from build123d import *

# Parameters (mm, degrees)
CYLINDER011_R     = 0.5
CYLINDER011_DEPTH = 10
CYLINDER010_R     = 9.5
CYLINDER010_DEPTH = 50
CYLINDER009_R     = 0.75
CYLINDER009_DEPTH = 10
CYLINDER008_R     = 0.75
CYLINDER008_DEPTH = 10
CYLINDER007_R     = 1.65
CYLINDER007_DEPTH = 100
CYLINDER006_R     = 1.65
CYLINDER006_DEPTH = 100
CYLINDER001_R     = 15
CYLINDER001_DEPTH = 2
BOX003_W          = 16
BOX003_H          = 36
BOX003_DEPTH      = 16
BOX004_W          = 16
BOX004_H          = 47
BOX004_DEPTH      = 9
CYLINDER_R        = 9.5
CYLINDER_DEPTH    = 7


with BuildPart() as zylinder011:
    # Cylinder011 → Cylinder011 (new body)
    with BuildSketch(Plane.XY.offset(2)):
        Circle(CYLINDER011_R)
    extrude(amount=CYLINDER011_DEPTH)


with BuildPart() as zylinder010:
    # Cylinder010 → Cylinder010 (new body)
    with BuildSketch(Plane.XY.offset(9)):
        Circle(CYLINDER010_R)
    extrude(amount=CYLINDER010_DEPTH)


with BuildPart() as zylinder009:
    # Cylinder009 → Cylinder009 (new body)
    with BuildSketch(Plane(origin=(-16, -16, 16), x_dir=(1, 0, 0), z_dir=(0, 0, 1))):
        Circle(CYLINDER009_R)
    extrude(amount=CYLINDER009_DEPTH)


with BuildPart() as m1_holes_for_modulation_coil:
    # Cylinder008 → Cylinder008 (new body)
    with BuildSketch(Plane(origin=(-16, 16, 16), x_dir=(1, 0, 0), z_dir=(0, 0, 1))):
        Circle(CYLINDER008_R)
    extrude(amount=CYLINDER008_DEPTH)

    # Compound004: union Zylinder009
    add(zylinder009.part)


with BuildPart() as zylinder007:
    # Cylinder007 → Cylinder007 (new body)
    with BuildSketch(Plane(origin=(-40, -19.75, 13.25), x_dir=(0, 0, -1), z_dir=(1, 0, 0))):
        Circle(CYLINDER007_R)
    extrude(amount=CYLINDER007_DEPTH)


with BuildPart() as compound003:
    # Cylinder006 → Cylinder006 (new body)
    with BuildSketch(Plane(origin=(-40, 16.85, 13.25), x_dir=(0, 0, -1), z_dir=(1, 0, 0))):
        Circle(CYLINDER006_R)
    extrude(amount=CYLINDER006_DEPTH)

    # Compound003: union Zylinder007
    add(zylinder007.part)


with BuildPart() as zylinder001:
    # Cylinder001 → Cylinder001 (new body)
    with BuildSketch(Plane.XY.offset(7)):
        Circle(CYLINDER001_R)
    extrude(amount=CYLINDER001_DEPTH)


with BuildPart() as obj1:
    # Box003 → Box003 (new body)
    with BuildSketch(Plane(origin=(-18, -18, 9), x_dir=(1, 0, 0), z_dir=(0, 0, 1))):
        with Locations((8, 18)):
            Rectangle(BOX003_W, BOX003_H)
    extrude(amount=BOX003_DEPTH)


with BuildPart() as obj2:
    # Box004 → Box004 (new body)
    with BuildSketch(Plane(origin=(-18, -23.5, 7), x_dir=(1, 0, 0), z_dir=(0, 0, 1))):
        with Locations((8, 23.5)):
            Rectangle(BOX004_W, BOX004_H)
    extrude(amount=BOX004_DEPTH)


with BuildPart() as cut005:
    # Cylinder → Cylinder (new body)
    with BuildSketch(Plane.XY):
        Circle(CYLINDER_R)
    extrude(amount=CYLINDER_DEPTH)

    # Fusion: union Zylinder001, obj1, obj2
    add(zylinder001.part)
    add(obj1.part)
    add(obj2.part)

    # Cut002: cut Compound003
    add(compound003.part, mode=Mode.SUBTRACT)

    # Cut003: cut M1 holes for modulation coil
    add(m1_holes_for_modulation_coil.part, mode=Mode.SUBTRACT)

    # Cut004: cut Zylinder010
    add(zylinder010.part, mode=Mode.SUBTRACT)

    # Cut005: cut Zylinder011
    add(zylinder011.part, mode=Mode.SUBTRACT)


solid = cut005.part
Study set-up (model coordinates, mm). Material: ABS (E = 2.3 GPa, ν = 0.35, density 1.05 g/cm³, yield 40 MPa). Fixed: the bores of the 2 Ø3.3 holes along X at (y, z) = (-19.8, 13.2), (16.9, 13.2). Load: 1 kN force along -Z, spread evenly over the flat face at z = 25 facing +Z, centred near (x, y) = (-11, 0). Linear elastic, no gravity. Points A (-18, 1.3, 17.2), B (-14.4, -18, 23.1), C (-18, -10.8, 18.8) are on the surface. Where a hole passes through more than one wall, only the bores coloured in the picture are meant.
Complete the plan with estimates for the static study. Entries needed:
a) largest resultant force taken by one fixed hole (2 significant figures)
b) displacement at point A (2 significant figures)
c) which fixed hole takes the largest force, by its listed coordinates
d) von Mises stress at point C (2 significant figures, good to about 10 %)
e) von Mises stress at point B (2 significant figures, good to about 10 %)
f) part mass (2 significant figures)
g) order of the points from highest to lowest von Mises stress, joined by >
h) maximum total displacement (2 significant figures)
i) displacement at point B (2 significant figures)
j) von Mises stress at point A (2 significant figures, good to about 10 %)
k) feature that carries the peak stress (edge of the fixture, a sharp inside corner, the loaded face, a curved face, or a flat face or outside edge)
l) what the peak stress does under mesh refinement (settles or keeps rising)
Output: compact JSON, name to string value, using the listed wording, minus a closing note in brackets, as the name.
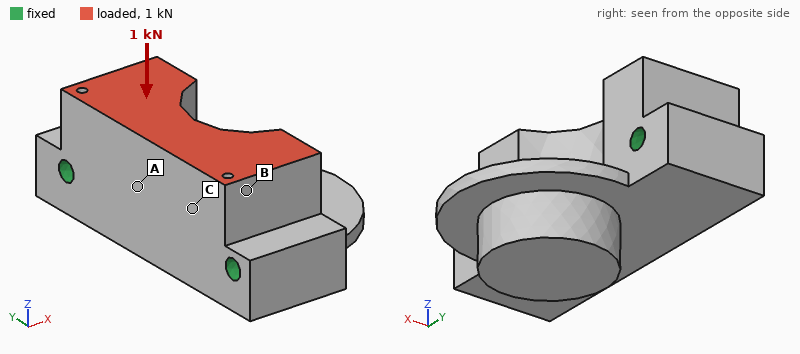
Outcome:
{"largest resultant force taken by one fixed hole": "550 N", "displacement at point A": "57 µm", "which fixed hole takes the largest force, by its listed coordinates": "(16.9, 13.2)", "von Mises stress at point C": "4.2 MPa", "von Mises stress at point B": "2.3 MPa", "part mass": "13 g", "order of the points from highest to lowest von Mises stress, joined by >": "C > B > A", "maximum total displacement": "66 µm", "displacement at point B": "28 µm", "von Mises stress at point A": "1.4 MPa", "feature that carries the peak stress": "edge of the fixture", "what the peak stress does under mesh refinement": "keeps rising"}
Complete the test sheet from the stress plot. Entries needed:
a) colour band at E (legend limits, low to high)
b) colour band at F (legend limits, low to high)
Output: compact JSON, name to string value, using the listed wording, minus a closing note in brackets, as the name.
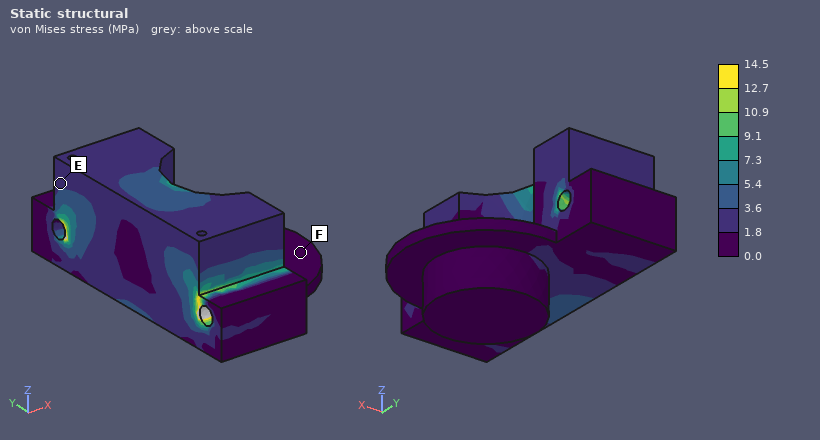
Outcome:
{"colour band at E": "1.8 to 3.6 MPa", "colour band at F": "0.0 to 1.8 MPa"}
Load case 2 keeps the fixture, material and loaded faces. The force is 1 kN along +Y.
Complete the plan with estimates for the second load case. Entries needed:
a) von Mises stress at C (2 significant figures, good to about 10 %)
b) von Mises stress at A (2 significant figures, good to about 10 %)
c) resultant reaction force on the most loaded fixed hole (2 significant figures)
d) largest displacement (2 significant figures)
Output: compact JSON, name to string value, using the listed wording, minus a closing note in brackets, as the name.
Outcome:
{"von Mises stress at C": "4.2 MPa", "von Mises stress at A": "2.9 MPa", "resultant reaction force on the most loaded fixed hole": "620 N", "largest displacement": "72 µm"}
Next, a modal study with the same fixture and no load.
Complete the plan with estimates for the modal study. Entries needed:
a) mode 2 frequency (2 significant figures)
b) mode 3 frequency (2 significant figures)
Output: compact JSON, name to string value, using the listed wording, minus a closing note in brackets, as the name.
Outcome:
{"mode 2 frequency": "6900 Hz", "mode 3 frequency": "7100 Hz"}
